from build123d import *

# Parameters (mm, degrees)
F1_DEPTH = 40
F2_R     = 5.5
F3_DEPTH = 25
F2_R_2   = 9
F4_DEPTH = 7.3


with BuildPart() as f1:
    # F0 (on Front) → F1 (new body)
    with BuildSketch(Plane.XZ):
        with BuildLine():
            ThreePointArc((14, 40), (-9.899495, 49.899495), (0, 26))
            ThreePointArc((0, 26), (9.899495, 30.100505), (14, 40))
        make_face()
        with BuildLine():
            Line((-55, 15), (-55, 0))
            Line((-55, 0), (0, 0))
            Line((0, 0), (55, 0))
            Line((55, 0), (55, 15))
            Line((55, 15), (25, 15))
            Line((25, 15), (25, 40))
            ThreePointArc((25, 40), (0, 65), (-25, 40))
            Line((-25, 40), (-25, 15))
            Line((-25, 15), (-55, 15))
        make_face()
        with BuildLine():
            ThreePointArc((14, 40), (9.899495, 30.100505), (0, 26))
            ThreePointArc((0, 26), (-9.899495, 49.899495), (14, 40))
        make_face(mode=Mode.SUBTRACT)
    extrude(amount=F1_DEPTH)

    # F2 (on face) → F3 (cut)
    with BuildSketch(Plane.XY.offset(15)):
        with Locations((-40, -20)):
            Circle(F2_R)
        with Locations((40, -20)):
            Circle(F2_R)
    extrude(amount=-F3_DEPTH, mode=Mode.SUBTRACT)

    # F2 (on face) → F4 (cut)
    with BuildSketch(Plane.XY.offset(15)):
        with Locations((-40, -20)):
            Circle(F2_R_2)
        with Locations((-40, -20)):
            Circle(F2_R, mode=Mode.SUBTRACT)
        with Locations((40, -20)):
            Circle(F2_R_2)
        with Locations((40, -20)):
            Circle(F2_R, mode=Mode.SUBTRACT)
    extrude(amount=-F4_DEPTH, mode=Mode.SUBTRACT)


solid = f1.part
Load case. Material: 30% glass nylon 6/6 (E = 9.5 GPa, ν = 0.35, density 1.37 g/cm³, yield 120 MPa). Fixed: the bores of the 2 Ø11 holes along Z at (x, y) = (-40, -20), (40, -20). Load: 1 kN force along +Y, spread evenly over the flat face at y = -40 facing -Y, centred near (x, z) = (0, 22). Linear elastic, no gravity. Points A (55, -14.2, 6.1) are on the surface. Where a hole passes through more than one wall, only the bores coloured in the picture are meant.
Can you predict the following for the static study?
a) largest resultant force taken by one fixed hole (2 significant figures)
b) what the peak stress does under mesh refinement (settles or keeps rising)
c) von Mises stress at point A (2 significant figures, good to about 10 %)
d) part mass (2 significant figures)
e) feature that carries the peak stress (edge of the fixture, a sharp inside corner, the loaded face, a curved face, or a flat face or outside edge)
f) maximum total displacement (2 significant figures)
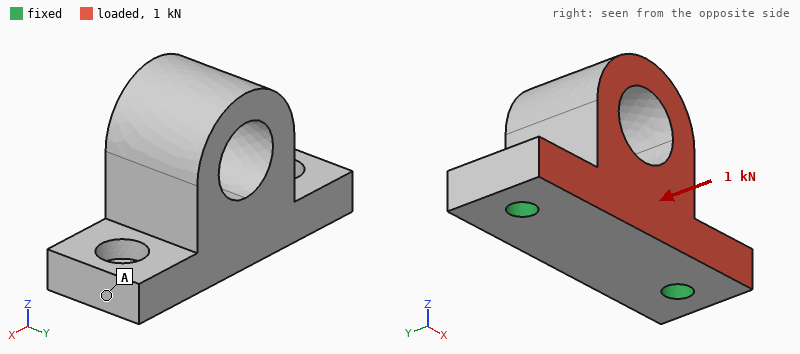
500 N
keeps rising
2.4 MPa
170 g
edge of the fixture
0.16 mm
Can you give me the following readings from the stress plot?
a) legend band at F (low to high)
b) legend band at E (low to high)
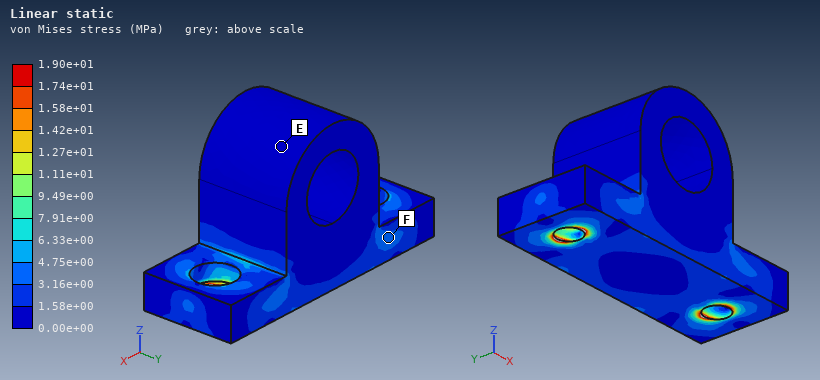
3.16e+00 to 4.75e+00 MPa
0.00e+00 to 1.58e+00 MPa
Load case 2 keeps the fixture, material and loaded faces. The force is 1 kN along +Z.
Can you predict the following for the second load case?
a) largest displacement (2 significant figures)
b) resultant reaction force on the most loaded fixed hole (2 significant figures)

0.16 mm
560 N
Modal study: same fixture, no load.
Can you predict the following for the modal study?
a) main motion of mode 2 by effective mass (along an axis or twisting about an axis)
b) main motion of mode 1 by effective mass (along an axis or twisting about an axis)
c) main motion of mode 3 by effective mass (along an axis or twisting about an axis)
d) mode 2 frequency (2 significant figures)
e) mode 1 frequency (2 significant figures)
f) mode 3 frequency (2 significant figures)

along X
along Y
along Z
3100 Hz
1200 Hz
3600 Hz
